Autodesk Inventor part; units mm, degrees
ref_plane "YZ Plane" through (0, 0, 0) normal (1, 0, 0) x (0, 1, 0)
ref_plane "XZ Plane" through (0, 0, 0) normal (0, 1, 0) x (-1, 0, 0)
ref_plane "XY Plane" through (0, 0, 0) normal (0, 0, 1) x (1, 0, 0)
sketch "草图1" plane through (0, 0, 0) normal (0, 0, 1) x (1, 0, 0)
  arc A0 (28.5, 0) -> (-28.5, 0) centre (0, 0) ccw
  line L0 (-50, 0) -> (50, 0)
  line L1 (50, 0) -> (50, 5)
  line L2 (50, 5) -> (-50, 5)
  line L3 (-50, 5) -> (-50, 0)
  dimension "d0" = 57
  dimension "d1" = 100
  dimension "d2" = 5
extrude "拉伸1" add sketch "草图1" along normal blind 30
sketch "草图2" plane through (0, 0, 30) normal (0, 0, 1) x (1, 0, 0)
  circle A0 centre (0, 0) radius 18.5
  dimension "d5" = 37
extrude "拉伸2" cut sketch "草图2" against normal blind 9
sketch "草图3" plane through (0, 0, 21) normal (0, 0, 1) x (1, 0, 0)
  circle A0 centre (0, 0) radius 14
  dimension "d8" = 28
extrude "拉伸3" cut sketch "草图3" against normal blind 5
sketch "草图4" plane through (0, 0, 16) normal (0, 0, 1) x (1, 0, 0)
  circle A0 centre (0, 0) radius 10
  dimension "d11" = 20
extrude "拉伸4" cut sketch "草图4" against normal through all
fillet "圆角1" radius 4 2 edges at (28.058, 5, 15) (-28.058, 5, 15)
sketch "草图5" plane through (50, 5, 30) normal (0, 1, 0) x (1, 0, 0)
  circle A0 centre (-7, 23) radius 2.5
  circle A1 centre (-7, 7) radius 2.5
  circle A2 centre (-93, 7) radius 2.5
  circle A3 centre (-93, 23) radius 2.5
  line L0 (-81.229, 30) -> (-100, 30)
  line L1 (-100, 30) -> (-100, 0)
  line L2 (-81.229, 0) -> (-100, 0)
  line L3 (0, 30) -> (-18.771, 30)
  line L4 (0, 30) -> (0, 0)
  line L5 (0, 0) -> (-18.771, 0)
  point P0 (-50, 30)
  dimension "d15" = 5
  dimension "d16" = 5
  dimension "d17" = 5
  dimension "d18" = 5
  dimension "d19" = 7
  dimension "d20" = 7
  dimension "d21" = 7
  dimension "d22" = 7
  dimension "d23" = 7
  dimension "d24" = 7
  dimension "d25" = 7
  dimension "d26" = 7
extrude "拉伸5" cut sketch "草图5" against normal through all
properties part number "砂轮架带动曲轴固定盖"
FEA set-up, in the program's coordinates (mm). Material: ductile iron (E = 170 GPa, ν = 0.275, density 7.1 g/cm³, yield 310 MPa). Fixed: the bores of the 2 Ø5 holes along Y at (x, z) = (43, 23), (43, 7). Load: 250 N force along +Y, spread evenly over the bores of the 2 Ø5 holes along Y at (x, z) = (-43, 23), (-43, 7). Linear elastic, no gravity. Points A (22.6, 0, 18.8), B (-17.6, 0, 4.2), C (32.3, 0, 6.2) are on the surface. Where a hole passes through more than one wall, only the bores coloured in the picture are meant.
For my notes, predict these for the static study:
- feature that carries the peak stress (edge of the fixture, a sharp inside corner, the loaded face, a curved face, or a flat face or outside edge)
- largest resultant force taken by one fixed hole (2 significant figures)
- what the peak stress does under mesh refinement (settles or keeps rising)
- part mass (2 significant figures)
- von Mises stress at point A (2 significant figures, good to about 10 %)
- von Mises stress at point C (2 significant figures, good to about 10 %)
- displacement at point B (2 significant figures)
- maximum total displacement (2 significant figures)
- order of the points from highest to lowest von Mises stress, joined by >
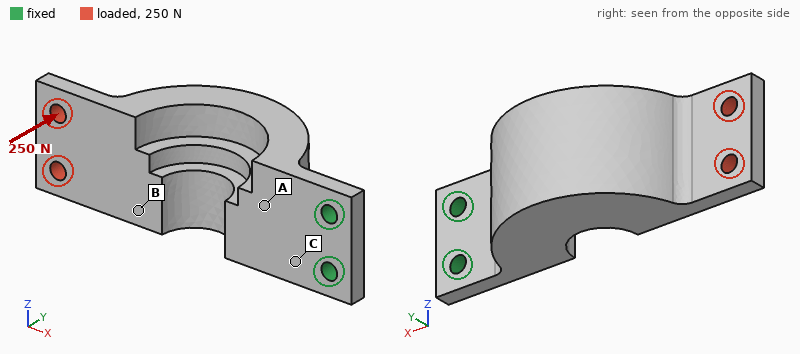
edge of the fixture
130 N
keeps rising
250 g
35 MPa
140 MPa
0.29 mm
0.49 mm
C > A > B
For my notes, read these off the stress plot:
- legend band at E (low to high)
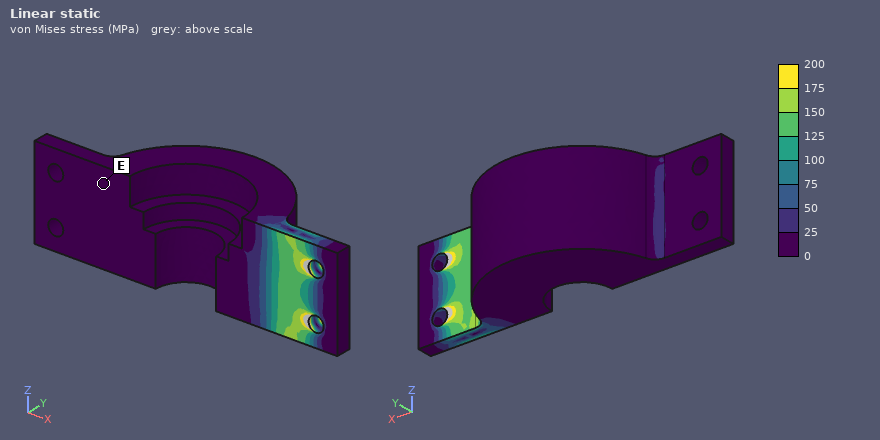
0 to 25 MPa
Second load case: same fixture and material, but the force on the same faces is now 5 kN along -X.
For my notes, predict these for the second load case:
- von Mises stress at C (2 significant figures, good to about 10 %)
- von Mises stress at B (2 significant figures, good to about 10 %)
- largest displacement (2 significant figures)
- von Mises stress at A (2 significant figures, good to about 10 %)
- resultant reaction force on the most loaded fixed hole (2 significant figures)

40 MPa
25 MPa
0.14 mm
51 MPa
2.5 kN
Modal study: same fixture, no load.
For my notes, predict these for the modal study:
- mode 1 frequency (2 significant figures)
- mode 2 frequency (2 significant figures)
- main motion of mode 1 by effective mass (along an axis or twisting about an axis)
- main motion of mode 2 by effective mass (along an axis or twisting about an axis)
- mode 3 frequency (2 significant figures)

440 Hz
1800 Hz
along Y
along Z
2600 Hz
